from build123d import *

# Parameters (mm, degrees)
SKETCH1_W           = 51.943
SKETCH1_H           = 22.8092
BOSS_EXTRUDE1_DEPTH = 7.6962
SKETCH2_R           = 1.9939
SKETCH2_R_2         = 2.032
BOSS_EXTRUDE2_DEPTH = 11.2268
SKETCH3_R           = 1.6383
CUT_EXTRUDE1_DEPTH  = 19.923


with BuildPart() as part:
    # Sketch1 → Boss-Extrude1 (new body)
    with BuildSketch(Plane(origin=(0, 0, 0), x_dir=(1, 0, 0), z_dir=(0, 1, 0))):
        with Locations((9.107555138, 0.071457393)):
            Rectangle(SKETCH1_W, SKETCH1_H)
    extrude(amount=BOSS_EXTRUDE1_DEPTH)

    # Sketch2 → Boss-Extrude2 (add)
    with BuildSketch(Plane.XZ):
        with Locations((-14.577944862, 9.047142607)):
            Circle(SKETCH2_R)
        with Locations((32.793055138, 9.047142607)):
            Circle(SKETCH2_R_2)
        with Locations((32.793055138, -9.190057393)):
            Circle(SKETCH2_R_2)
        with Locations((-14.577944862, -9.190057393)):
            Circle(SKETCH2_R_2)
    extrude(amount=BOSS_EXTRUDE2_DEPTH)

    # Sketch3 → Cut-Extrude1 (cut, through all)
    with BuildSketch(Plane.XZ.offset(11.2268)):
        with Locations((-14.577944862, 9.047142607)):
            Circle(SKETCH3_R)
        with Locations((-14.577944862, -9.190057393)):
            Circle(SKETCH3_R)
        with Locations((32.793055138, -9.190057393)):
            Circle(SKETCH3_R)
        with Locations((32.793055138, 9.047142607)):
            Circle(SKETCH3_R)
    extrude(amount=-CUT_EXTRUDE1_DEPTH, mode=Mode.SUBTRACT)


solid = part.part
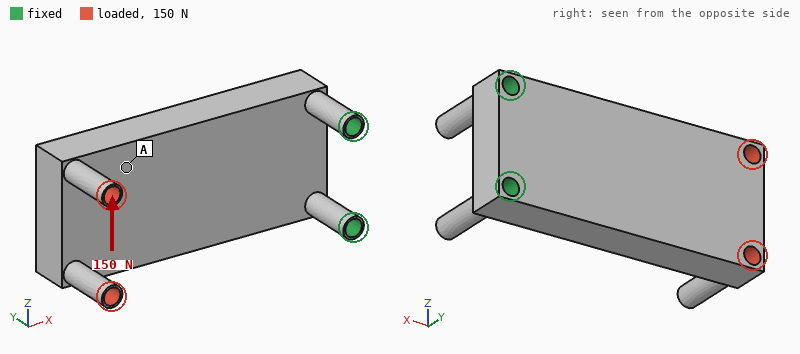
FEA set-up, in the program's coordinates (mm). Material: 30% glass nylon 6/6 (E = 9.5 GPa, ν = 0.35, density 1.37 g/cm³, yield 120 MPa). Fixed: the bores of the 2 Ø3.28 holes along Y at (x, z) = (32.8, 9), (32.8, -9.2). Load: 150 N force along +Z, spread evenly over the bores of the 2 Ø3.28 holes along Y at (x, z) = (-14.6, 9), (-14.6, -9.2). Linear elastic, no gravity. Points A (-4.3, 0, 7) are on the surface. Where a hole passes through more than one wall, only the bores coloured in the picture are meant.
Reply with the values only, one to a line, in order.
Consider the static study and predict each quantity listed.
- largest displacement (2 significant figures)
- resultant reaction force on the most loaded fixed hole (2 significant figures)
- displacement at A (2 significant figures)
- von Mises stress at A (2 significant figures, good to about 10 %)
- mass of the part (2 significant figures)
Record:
0.36 mm
390 N
0.072 mm
5.4 MPa
12 g
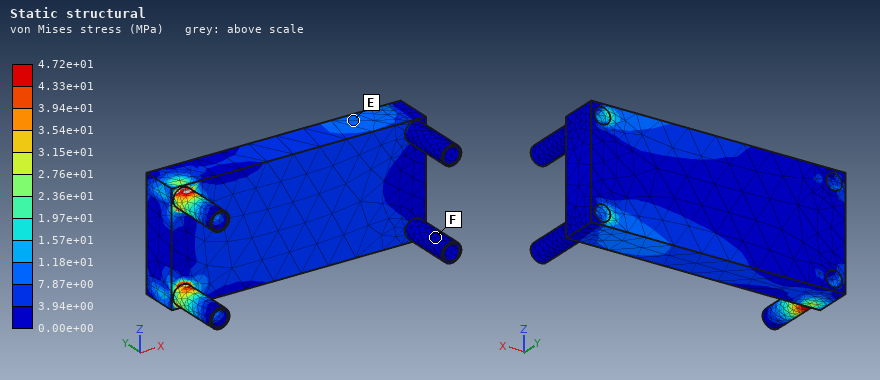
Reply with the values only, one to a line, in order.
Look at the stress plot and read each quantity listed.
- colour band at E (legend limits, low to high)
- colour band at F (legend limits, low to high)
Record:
7.87e+00 to 1.18e+01 MPa
0.00e+00 to 3.94e+00 MPa
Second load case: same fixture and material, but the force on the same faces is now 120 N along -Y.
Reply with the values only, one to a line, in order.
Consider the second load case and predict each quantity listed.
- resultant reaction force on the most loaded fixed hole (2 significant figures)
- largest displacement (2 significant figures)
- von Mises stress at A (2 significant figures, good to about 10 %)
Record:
60 N
0.67 mm
5.6 MPa
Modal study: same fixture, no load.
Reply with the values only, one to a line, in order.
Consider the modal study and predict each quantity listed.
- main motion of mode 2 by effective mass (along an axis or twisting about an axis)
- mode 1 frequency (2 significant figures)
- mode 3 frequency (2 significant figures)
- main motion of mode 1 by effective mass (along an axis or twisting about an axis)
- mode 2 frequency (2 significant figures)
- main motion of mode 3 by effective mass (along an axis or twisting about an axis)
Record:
along Z
1200 Hz
4900 Hz
along Y
3500 Hz
twisting about X
